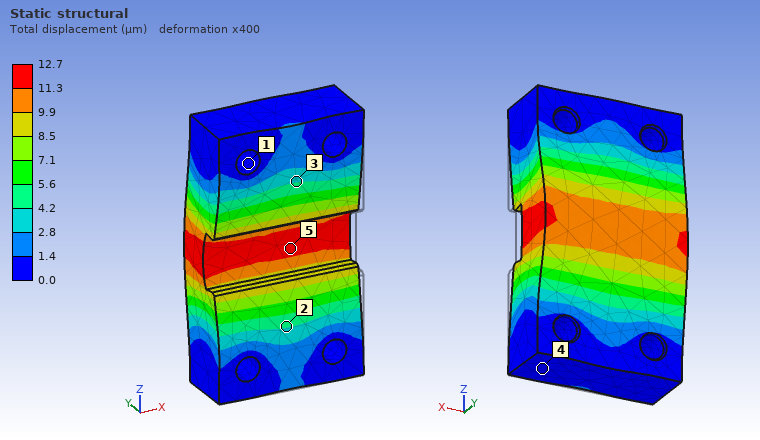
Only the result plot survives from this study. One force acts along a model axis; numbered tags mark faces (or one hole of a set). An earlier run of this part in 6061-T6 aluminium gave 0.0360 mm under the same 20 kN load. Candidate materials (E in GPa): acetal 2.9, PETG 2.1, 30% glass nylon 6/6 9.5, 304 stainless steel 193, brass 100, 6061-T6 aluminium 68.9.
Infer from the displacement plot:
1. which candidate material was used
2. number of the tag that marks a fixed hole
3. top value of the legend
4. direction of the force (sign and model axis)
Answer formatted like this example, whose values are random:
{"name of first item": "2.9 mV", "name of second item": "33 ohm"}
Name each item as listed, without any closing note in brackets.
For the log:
{"which candidate material was used": "304 stainless steel", "number of the tag that marks a fixed hole": "1", "top value of the legend": "12.7 µm", "direction of the force": "+Y"}
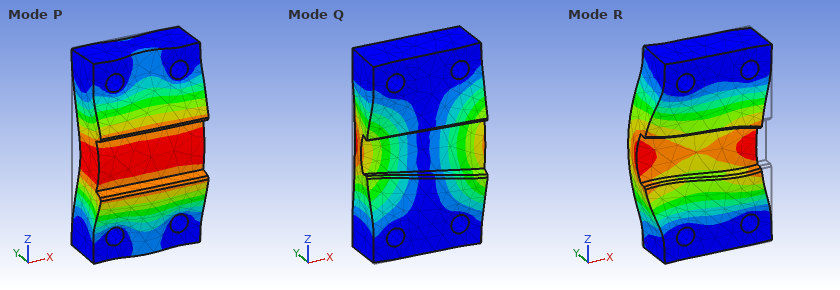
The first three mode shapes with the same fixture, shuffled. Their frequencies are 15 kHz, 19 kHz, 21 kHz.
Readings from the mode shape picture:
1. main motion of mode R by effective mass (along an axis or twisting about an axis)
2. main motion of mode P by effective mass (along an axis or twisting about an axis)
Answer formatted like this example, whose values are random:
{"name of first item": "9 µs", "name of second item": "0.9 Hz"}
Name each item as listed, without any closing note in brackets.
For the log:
{"main motion of mode R by effective mass": "along X", "main motion of mode P by effective mass": "along Y"}
